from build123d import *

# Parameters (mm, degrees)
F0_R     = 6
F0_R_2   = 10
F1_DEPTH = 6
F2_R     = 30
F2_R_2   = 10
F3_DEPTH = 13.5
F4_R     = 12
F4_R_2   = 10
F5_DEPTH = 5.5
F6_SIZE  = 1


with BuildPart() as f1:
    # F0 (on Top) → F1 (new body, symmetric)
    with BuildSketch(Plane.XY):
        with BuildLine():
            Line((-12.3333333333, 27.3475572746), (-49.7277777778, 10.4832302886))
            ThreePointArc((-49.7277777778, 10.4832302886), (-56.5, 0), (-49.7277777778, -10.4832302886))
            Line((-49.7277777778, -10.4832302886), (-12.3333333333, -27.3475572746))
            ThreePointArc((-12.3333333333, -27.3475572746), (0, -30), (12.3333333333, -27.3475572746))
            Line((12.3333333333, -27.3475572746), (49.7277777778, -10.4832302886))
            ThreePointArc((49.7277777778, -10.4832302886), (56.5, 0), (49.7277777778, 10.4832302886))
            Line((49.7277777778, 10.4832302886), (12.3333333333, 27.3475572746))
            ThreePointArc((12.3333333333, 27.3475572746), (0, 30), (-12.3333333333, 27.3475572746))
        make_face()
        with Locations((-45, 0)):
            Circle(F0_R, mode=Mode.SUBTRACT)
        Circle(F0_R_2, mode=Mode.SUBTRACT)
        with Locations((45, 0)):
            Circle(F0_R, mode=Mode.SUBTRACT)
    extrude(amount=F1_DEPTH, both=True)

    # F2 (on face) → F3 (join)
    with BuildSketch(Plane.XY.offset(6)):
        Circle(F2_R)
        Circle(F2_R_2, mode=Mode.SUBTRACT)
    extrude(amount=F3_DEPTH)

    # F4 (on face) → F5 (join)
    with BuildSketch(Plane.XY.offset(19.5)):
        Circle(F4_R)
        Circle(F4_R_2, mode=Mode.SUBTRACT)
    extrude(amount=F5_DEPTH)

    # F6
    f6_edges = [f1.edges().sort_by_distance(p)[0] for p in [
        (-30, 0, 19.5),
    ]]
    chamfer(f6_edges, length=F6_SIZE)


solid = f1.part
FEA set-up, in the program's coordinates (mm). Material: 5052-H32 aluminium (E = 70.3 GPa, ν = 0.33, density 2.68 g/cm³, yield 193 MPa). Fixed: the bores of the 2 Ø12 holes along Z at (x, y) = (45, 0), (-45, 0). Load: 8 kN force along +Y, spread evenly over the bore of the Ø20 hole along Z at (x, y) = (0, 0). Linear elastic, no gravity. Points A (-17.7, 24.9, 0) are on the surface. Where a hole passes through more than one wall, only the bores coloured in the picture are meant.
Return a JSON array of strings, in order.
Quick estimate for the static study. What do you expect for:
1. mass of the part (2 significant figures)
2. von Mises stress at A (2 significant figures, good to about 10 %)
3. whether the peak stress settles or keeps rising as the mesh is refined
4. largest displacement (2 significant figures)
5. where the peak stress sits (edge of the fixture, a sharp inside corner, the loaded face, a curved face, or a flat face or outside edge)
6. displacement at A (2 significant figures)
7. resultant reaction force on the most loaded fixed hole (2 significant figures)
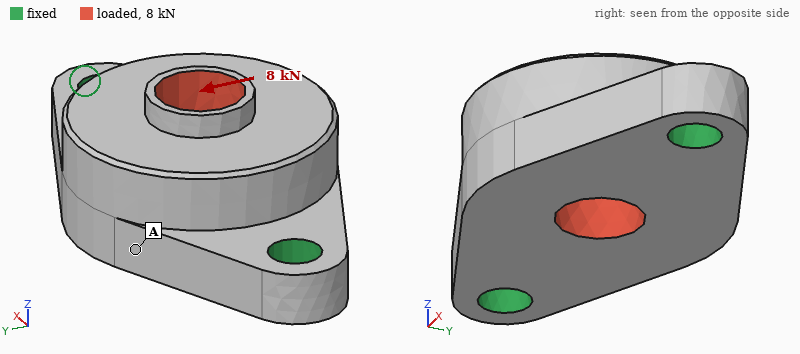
["220 g", "14 MPa", "keeps rising", "56 µm", "edge of the fixture", "34 µm", "4.0 kN"]
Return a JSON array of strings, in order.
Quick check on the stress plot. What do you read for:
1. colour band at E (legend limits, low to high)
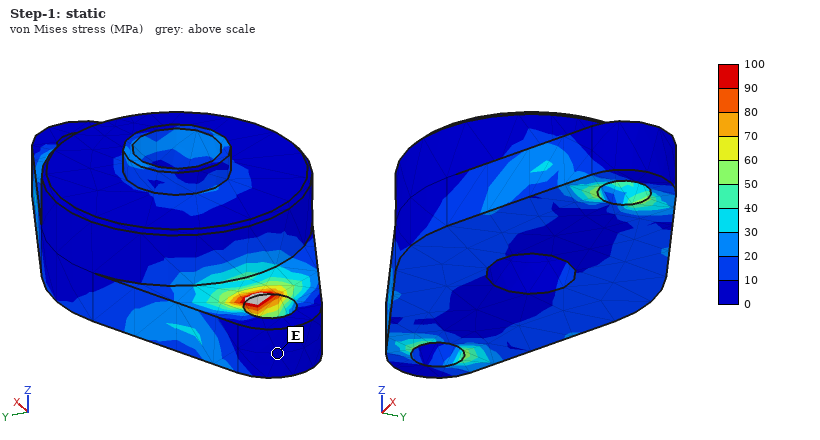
["0 to 10 MPa"]
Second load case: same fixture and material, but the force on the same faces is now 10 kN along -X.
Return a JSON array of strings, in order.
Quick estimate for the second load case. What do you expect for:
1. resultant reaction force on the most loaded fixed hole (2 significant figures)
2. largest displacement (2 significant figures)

["5.2 kN", "15 µm"]
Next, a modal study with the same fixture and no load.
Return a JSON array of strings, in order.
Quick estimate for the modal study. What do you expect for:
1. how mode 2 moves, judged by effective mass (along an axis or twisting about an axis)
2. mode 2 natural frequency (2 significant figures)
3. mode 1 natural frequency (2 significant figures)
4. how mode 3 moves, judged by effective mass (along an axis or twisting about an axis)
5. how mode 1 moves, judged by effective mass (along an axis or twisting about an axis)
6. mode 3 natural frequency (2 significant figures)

["along Z", "7100 Hz", "4700 Hz", "along Y", "along Y", "11 kHz"]
